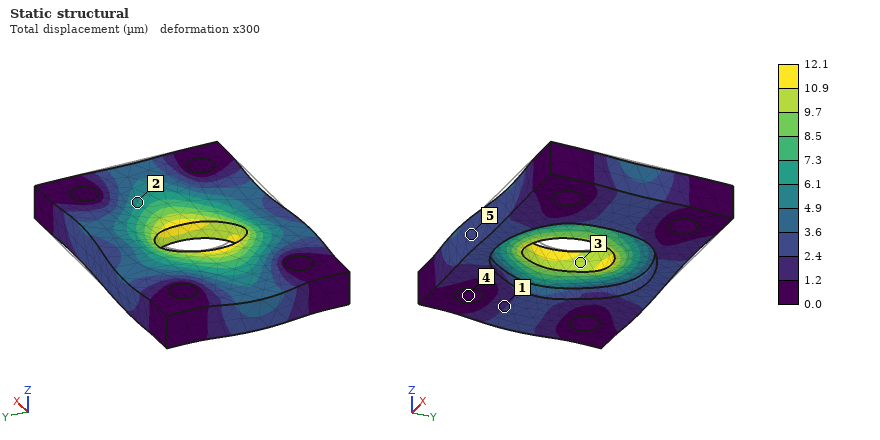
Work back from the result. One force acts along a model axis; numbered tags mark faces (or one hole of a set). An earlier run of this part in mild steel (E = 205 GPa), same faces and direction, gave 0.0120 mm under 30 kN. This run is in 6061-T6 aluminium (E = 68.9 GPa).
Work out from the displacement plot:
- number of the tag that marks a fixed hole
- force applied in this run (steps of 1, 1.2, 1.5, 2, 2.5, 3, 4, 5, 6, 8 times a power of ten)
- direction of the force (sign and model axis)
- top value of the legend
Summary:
4
10 kN
-X
12.1 µm
